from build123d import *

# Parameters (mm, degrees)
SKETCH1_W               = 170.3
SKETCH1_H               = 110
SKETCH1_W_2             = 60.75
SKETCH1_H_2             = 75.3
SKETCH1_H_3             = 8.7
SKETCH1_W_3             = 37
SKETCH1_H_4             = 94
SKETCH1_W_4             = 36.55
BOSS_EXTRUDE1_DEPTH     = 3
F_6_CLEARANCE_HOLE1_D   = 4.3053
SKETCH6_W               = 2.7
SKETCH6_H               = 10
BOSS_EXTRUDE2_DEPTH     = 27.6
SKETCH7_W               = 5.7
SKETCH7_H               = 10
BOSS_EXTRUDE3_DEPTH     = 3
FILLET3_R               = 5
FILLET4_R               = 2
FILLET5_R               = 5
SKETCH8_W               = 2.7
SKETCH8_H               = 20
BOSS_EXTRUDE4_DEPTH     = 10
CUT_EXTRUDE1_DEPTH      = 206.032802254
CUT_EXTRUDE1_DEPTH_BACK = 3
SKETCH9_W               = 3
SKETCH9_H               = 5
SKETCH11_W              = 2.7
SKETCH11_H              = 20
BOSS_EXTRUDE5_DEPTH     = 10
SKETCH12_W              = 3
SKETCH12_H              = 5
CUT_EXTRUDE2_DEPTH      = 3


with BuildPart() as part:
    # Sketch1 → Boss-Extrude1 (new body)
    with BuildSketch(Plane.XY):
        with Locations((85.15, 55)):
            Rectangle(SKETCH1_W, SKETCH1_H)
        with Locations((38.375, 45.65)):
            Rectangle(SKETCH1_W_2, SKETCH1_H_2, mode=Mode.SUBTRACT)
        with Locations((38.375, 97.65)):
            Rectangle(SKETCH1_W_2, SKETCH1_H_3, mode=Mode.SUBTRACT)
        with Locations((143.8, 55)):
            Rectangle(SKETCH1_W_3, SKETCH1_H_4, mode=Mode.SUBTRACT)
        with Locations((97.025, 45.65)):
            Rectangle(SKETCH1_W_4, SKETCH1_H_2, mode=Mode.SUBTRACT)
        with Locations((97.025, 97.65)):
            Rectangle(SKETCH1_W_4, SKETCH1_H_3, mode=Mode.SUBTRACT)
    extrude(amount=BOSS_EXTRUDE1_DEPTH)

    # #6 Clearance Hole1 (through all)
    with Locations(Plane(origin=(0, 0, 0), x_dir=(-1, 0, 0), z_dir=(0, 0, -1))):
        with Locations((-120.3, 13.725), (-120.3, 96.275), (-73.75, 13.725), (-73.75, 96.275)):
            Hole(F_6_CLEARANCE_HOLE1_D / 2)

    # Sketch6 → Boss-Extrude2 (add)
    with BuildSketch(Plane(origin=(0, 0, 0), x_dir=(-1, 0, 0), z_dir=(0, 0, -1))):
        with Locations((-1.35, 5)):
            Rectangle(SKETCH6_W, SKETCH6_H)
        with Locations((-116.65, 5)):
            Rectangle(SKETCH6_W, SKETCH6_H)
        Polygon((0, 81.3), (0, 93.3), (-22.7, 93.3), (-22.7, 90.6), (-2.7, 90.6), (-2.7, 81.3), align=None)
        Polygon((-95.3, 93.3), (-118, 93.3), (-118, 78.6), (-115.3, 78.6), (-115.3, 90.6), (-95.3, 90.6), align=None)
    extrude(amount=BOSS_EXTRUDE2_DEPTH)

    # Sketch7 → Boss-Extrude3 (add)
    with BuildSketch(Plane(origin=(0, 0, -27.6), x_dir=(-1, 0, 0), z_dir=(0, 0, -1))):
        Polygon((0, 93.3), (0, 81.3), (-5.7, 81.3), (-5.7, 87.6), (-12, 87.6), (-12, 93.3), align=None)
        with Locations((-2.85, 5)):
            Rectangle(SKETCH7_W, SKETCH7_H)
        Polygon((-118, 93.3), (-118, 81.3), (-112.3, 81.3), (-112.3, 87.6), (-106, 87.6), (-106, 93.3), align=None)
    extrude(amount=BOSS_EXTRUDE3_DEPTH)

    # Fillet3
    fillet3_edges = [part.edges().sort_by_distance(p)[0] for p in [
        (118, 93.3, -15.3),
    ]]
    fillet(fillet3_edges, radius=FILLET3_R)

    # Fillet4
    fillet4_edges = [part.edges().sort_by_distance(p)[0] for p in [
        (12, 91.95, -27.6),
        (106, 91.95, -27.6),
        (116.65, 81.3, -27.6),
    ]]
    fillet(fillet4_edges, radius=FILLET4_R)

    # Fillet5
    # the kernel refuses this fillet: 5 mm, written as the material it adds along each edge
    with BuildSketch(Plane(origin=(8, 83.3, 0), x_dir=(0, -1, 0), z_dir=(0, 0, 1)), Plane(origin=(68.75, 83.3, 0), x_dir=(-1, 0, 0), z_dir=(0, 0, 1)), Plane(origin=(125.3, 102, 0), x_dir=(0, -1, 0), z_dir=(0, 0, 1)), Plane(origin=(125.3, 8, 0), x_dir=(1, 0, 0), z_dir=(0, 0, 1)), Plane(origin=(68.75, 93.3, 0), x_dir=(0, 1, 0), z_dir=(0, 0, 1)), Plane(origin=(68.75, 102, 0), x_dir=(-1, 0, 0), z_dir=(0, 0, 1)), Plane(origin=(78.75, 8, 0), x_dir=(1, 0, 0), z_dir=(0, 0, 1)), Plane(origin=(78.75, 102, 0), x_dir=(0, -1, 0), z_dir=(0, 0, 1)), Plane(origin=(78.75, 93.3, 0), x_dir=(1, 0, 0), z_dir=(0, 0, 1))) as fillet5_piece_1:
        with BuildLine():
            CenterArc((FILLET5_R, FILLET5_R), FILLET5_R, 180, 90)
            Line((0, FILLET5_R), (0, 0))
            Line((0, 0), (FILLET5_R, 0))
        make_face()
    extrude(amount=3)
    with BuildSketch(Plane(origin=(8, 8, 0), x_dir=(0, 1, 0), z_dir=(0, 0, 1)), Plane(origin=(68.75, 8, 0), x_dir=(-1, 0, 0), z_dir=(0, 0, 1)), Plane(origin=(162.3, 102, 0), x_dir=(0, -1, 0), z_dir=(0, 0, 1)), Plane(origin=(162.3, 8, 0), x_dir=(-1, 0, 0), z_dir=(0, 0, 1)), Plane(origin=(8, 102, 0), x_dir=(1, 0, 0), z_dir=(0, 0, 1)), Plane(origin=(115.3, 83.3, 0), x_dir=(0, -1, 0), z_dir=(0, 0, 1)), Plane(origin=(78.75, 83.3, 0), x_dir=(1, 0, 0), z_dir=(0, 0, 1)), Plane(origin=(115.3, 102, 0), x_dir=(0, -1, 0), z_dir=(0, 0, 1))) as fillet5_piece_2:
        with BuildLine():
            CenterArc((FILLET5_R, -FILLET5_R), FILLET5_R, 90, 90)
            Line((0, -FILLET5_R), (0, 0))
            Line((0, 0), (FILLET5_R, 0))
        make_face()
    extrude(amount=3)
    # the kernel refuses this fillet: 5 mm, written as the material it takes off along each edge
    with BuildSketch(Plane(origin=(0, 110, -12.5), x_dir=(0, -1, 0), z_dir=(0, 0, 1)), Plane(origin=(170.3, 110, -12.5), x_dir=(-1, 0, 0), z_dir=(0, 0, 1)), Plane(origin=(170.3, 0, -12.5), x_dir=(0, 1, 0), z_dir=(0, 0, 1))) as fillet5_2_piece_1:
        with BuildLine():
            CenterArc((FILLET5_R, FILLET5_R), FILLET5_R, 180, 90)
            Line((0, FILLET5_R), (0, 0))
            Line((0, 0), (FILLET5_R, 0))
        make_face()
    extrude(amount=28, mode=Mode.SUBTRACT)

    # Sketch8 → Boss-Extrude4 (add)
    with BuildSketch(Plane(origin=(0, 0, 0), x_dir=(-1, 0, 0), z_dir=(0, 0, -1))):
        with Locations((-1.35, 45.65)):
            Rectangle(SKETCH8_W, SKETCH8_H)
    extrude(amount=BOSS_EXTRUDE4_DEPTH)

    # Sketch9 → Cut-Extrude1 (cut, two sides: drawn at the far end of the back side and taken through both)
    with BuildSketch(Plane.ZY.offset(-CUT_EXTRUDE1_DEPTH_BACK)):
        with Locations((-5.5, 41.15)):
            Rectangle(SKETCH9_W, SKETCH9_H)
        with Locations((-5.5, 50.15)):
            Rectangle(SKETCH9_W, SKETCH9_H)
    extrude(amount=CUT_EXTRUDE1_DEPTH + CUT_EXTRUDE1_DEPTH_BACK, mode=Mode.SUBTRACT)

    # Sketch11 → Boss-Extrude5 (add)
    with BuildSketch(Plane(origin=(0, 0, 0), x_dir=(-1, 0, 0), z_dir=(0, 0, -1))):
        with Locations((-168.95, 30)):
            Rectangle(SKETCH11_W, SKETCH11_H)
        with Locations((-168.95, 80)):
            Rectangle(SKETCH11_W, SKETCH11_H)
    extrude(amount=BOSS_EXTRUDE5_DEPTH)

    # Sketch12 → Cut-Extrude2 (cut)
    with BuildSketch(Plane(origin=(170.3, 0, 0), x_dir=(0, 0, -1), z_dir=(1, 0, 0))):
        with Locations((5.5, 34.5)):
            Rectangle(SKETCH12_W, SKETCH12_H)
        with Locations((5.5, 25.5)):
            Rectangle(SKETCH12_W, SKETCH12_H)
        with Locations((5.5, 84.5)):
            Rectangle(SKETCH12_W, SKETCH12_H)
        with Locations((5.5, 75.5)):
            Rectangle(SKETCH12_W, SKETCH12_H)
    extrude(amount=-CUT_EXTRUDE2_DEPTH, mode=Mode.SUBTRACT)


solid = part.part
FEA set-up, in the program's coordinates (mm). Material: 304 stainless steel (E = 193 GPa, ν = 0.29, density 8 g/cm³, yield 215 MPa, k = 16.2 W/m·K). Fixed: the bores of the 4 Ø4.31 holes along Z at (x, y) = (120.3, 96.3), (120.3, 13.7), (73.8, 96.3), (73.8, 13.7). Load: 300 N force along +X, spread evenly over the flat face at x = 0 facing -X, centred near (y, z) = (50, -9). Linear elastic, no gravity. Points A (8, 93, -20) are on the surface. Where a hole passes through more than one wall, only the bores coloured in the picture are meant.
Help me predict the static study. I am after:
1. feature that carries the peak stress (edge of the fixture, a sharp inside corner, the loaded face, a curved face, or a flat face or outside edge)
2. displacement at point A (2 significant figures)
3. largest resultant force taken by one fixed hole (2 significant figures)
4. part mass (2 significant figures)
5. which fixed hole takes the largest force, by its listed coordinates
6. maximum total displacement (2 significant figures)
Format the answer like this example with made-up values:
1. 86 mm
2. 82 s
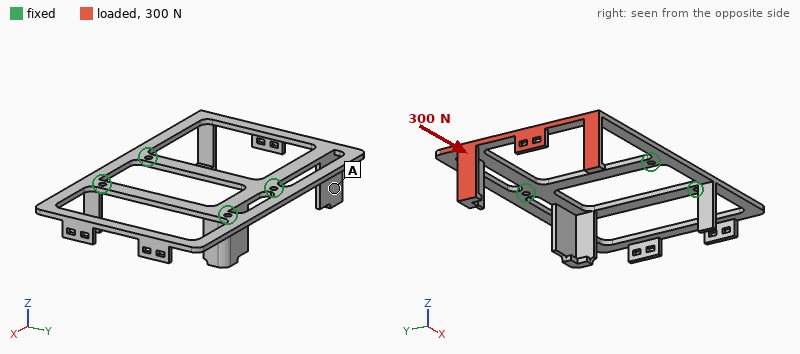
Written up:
1. a curved face
2. 0.66 mm
3. 130 N
4. 240 g
5. (73.8, 96.3)
6. 1.2 mm
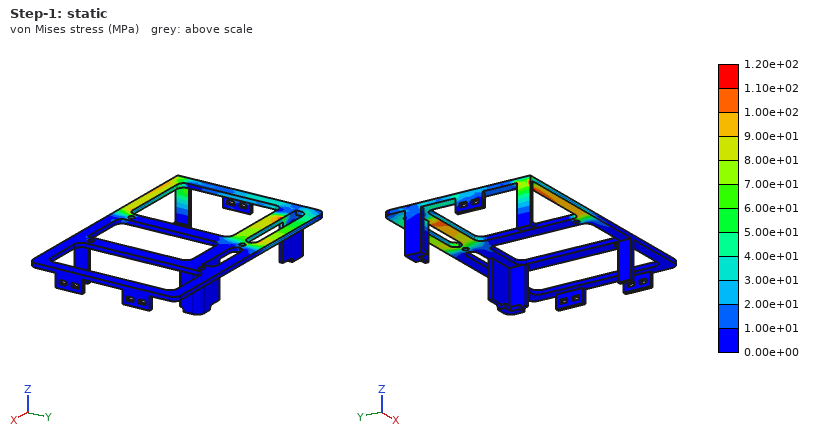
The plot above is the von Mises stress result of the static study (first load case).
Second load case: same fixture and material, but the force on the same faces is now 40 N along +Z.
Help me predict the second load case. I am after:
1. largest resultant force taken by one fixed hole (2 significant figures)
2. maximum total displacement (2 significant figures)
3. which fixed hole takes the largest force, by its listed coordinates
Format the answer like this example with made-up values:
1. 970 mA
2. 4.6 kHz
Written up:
1. 31 N
2. 0.65 mm
3. (73.8, 96.3)
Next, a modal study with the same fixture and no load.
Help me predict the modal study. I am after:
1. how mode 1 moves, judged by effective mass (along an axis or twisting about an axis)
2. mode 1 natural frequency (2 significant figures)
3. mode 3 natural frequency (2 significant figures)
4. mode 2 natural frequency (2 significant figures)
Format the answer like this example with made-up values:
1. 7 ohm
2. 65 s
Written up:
1. along Z
2. 200 Hz
3. 380 Hz
4. 370 Hz
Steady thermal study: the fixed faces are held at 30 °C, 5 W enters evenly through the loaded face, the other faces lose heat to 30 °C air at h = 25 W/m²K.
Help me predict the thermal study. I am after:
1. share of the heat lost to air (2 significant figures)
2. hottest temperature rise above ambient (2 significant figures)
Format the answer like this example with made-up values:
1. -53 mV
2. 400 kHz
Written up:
1. 96 %
2. 56 K
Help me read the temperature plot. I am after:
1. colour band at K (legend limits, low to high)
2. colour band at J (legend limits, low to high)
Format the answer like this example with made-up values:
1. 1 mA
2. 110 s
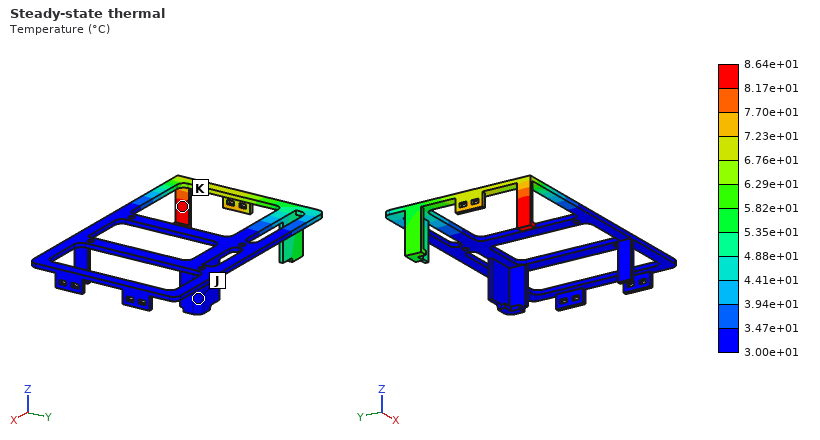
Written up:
1. 8.17e+01 to 8.64e+01 °C
2. 3.00e+01 to 3.47e+01 °C
